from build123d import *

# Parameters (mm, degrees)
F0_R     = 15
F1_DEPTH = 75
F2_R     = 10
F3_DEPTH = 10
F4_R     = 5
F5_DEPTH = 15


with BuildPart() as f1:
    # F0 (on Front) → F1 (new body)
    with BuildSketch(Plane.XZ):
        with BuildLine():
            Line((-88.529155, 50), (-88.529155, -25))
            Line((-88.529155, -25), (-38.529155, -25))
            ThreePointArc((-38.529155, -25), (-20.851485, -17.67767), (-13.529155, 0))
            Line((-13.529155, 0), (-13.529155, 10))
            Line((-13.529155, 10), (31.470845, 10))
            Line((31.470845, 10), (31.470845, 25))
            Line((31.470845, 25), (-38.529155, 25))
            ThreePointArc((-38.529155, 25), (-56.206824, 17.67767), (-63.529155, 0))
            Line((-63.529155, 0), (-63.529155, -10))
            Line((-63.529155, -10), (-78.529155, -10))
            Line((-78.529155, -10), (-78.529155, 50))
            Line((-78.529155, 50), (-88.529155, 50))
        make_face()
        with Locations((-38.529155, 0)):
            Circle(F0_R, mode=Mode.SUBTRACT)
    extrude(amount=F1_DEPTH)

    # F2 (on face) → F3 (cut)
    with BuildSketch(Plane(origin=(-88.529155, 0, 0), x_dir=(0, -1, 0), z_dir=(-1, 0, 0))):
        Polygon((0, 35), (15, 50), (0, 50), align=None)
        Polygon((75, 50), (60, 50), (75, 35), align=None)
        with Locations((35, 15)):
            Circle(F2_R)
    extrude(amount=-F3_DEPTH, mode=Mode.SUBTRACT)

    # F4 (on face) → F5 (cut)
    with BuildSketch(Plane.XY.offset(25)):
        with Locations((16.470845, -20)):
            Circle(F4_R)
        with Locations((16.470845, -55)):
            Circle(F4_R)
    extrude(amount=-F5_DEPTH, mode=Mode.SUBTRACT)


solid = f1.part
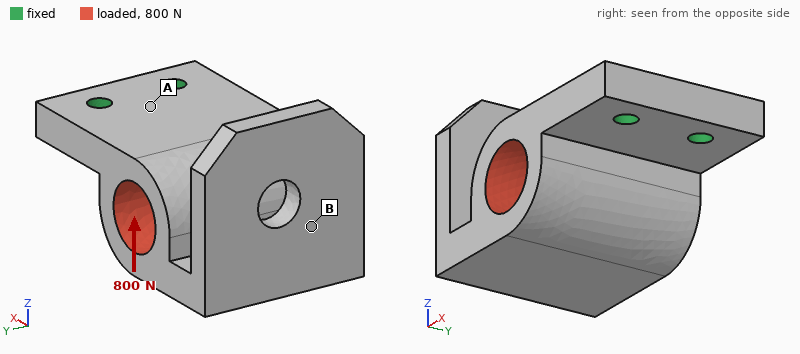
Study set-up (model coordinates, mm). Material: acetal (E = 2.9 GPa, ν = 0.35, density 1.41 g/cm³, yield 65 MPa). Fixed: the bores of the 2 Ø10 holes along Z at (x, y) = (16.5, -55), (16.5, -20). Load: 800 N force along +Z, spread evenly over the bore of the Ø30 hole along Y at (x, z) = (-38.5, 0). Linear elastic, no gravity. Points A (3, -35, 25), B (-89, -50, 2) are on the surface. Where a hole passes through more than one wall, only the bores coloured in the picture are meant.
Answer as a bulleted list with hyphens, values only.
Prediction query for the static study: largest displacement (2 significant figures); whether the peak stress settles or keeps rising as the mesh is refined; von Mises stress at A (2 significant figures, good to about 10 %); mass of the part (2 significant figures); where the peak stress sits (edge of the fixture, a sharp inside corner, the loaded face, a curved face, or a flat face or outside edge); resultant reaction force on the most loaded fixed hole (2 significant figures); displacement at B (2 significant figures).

- 1.8 mm
- keeps rising
- 9.5 MPa
- 320 g
- edge of the fixture
- 400 N
- 1.6 mm
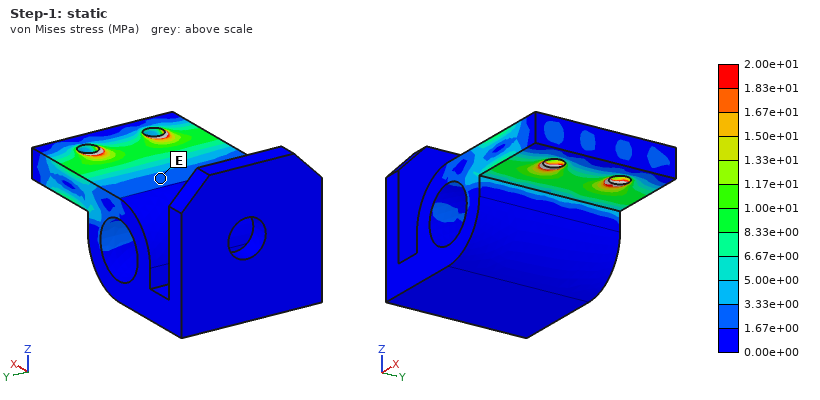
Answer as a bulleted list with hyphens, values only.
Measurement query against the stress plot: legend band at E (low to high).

- 1.67e+00 to 3.33e+00 MPa
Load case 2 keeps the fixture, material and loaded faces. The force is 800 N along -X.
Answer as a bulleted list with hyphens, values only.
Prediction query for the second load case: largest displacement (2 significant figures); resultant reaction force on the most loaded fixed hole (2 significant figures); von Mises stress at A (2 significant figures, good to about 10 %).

- 0.85 mm
- 400 N
- 3.5 MPa
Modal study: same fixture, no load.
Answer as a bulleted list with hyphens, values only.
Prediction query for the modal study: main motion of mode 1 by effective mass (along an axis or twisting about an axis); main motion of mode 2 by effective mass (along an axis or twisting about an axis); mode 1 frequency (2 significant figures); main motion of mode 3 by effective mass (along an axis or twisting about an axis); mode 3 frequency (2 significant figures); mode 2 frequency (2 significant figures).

- along Z
- along X
- 200 Hz
- along Y
- 540 Hz
- 470 Hz
